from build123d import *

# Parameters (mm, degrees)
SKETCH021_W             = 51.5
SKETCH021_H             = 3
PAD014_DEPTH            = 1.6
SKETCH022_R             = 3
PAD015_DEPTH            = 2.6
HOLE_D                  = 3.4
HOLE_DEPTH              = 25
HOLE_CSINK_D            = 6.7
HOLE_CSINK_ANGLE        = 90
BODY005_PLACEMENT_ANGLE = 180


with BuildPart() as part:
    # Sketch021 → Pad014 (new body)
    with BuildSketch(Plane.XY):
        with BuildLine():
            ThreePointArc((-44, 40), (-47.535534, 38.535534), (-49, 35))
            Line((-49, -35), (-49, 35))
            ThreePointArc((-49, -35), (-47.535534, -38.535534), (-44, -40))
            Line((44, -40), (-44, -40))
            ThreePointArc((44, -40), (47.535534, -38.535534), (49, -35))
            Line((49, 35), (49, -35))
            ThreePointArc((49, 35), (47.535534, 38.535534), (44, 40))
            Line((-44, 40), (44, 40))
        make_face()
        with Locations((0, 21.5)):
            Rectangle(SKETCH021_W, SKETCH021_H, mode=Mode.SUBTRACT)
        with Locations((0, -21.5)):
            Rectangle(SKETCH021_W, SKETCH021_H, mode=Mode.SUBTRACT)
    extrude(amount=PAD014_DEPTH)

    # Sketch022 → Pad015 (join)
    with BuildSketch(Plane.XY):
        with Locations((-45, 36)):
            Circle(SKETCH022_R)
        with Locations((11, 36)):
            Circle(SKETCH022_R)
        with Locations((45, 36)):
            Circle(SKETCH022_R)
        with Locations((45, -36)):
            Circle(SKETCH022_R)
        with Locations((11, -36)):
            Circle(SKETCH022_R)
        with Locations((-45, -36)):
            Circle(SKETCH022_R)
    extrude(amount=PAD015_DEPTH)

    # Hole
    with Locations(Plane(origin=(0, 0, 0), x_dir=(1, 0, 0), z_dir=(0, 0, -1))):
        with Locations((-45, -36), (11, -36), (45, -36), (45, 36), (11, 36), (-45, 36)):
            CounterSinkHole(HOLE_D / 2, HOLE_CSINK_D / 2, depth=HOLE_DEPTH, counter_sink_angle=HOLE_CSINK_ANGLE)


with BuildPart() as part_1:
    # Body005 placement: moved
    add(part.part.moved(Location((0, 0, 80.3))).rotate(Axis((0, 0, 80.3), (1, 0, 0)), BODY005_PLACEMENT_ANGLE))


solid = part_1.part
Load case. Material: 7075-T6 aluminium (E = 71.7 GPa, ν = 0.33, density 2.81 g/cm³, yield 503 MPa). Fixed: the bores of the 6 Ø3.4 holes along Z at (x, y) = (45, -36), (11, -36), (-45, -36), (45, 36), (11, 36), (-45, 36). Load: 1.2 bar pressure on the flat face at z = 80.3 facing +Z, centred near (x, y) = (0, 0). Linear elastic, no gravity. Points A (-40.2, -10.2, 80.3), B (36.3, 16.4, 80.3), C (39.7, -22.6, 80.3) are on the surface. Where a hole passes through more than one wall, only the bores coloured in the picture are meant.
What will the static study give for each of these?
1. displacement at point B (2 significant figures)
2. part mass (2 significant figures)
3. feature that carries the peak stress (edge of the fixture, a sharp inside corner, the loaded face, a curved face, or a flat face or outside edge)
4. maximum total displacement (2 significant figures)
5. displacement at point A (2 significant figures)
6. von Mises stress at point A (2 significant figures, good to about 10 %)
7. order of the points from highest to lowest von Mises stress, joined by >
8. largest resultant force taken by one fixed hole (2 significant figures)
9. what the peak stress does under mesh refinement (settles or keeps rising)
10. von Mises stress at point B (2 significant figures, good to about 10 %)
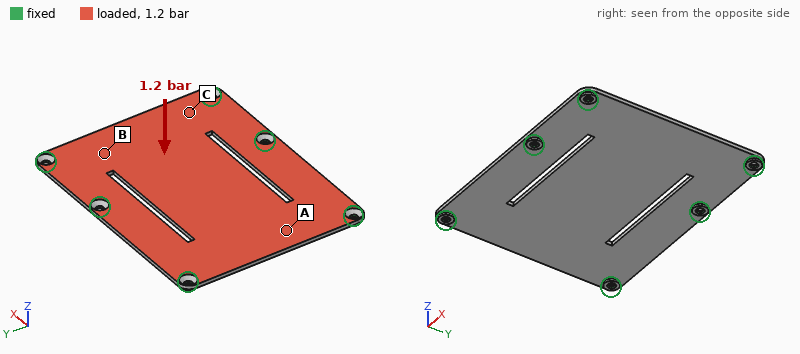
0.37 mm
34 g
edge of the fixture
1.0 mm
0.52 mm
77 MPa
A > B > C
430 N
keeps rising
48 MPa
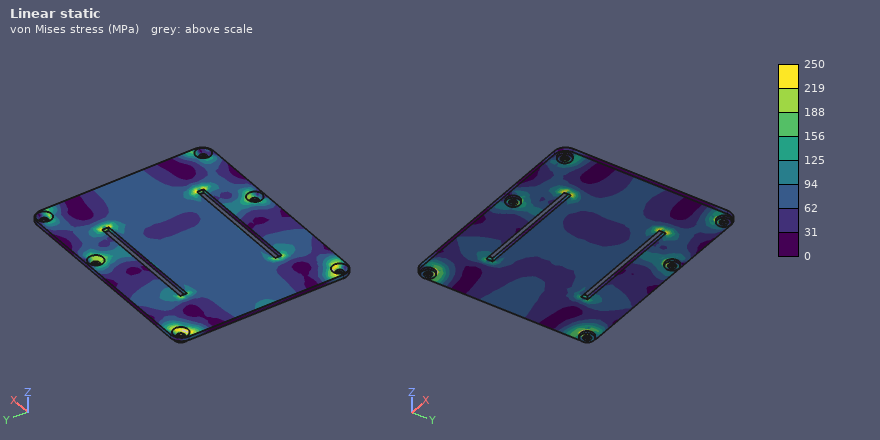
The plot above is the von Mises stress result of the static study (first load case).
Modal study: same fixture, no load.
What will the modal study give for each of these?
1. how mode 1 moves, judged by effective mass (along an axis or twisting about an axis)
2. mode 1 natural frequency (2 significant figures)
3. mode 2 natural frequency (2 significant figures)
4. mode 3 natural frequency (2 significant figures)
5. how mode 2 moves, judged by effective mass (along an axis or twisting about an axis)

along Z
980 Hz
1600 Hz
2000 Hz
twisting about Y
